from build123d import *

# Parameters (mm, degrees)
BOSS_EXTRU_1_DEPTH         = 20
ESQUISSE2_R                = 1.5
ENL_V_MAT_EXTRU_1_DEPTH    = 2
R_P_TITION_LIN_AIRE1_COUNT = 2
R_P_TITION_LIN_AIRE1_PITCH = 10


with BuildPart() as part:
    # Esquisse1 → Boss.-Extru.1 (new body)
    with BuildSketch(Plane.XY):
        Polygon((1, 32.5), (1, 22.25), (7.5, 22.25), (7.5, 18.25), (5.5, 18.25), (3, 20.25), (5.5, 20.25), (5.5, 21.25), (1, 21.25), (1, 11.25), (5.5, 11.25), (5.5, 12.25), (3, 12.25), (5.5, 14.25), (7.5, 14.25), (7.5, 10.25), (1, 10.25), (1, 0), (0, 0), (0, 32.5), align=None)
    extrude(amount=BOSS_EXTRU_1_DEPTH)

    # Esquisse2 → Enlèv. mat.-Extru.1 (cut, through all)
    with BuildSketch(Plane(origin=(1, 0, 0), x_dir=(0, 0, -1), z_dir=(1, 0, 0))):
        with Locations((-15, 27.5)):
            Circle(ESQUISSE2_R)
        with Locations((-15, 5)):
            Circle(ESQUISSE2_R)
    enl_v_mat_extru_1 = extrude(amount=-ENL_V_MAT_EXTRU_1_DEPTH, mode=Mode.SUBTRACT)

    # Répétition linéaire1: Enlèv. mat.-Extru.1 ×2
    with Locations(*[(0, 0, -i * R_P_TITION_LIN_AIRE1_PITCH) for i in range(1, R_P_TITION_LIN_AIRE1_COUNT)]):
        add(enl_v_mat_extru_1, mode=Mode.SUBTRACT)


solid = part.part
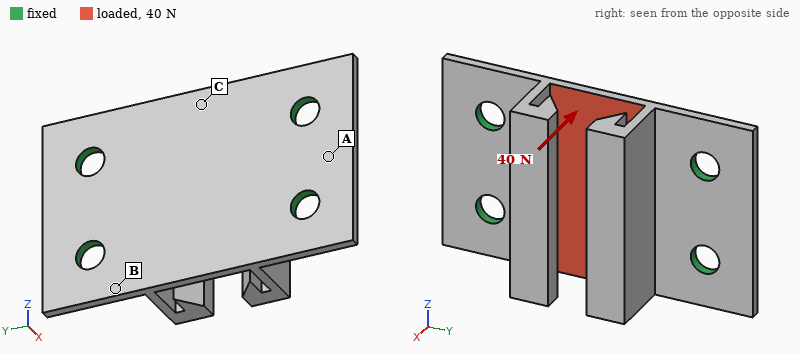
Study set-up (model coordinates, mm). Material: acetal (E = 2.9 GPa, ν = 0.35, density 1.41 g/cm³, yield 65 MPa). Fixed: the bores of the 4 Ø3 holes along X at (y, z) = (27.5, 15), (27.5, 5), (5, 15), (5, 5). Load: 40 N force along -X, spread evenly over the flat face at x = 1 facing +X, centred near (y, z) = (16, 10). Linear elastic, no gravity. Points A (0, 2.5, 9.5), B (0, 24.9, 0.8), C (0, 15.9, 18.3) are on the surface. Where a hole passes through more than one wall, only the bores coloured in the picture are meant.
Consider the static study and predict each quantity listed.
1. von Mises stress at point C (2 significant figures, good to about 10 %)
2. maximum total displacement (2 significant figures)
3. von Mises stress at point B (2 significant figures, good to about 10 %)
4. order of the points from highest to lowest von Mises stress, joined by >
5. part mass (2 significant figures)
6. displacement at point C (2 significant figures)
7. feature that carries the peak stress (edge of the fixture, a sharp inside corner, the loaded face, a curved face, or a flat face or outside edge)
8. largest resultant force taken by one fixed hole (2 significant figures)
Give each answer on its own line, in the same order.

18 MPa
0.44 mm
12 MPa
C > B > A
1.7 g
0.31 mm
a flat face or outside edge
10 N
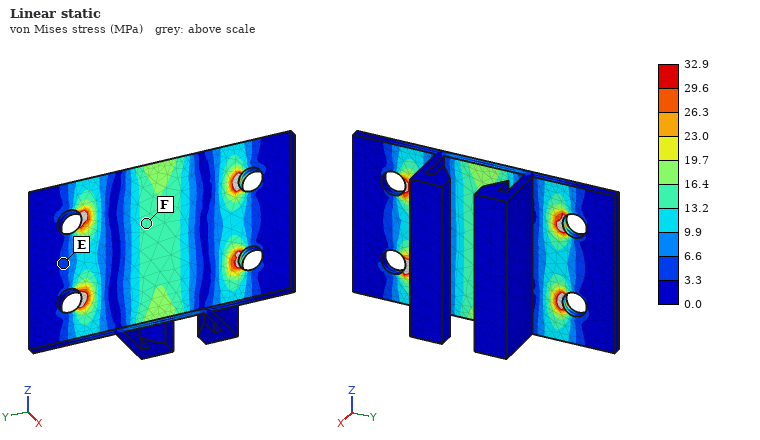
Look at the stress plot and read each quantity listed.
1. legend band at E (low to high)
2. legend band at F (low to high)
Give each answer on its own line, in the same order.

3.3 to 6.6 MPa
13.2 to 16.4 MPa
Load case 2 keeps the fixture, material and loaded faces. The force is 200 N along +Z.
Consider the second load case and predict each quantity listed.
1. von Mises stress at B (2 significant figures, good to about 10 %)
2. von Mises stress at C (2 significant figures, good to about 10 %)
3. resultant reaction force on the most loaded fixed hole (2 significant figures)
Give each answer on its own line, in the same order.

5.1 MPa
12 MPa
57 N
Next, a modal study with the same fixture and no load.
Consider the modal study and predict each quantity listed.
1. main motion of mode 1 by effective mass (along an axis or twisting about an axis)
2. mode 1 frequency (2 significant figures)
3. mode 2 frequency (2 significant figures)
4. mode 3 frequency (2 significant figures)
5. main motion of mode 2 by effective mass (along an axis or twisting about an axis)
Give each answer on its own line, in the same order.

along X
1400 Hz
2000 Hz
2400 Hz
along Y
